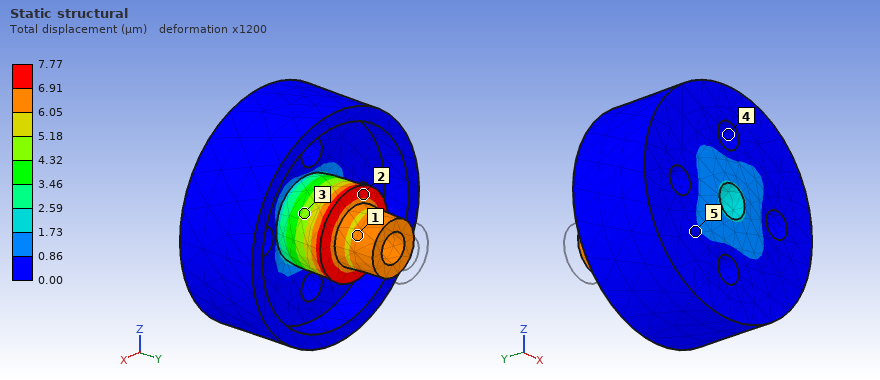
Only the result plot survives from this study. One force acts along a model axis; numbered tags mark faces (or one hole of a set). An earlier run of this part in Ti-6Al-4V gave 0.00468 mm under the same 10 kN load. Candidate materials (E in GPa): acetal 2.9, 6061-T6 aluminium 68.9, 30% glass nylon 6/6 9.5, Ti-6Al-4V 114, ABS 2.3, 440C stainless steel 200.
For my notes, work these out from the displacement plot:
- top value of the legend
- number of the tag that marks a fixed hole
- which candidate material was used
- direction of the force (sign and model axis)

7.77 µm
4
6061-T6 aluminium
-Y
